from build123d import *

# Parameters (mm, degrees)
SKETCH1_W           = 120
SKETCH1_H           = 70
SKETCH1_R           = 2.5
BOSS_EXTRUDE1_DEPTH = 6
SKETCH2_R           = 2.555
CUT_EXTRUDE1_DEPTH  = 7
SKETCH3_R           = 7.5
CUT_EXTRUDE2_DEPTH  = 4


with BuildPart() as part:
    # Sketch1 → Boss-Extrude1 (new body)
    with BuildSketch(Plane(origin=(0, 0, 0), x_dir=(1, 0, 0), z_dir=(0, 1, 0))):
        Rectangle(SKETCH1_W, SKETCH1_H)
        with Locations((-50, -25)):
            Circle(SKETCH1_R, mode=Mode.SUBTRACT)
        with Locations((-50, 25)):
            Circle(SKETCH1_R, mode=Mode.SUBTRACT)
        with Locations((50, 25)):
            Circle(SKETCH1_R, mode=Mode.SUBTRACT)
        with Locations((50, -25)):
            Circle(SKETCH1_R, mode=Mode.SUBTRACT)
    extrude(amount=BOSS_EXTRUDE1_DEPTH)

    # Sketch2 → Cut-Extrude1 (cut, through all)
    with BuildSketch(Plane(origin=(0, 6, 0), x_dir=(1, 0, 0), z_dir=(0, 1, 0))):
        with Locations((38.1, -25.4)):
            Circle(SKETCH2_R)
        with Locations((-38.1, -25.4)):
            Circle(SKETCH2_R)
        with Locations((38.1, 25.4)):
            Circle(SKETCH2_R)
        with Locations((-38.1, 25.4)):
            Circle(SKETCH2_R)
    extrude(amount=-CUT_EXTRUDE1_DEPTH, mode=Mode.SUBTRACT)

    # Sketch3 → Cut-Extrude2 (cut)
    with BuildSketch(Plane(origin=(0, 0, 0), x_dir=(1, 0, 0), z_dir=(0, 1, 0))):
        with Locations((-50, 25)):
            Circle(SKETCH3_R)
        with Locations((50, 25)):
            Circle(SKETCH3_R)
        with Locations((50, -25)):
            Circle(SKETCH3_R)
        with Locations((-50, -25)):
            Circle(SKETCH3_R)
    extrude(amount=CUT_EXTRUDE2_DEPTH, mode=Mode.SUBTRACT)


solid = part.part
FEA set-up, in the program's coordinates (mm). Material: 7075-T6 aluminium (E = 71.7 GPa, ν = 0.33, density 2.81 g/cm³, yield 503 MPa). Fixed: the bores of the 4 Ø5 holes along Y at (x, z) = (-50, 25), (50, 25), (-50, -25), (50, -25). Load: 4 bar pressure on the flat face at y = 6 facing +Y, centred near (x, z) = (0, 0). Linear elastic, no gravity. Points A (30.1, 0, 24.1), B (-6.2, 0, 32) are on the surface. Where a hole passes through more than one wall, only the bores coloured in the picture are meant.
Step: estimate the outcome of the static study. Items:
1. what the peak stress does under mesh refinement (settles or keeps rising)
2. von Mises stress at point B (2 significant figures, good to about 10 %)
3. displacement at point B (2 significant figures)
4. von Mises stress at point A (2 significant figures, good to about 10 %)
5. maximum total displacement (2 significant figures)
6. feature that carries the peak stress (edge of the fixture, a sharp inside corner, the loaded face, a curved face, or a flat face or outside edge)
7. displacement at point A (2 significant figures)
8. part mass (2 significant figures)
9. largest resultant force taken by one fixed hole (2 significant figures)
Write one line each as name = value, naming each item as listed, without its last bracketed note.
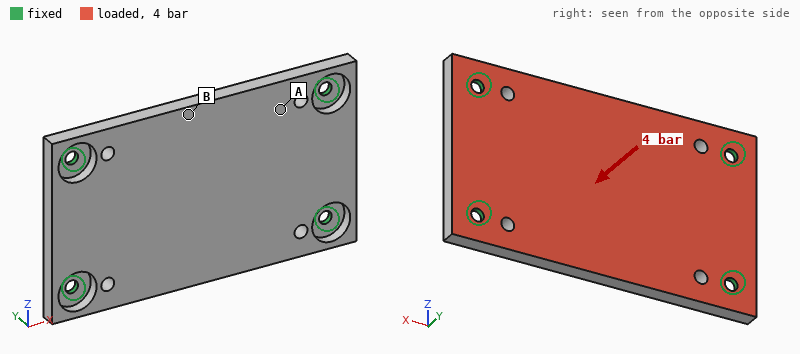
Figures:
what the peak stress does under mesh refinement = keeps rising
von Mises stress at point B = 53 MPa
displacement at point B = 0.19 mm
von Mises stress at point A = 23 MPa
maximum total displacement = 0.20 mm
feature that carries the peak stress = edge of the fixture
displacement at point A = 0.11 mm
part mass = 130 g
largest resultant force taken by one fixed hole = 1.7 kN
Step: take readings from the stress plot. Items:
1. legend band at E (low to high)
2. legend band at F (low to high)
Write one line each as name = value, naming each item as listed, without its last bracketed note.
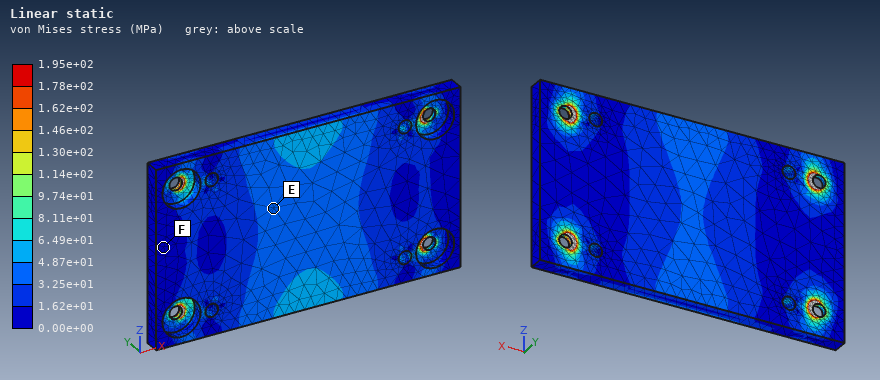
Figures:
legend band at E = 3.25e+01 to 4.87e+01 MPa
legend band at F = 0.00e+00 to 1.62e+01 MPa
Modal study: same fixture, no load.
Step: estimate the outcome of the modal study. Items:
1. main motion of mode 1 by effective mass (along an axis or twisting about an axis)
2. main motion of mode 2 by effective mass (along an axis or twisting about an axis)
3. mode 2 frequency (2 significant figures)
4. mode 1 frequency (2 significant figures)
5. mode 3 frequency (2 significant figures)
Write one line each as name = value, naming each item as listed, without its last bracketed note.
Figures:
main motion of mode 1 by effective mass = along Y
main motion of mode 2 by effective mass = twisting about X
mode 2 frequency = 3200 Hz
mode 1 frequency = 2000 Hz
mode 3 frequency = 5500 Hz
